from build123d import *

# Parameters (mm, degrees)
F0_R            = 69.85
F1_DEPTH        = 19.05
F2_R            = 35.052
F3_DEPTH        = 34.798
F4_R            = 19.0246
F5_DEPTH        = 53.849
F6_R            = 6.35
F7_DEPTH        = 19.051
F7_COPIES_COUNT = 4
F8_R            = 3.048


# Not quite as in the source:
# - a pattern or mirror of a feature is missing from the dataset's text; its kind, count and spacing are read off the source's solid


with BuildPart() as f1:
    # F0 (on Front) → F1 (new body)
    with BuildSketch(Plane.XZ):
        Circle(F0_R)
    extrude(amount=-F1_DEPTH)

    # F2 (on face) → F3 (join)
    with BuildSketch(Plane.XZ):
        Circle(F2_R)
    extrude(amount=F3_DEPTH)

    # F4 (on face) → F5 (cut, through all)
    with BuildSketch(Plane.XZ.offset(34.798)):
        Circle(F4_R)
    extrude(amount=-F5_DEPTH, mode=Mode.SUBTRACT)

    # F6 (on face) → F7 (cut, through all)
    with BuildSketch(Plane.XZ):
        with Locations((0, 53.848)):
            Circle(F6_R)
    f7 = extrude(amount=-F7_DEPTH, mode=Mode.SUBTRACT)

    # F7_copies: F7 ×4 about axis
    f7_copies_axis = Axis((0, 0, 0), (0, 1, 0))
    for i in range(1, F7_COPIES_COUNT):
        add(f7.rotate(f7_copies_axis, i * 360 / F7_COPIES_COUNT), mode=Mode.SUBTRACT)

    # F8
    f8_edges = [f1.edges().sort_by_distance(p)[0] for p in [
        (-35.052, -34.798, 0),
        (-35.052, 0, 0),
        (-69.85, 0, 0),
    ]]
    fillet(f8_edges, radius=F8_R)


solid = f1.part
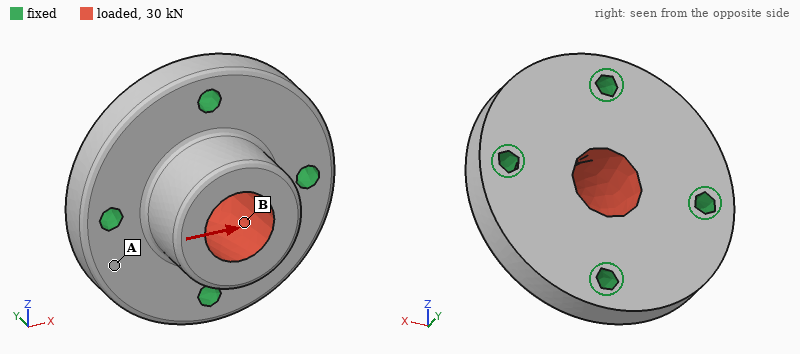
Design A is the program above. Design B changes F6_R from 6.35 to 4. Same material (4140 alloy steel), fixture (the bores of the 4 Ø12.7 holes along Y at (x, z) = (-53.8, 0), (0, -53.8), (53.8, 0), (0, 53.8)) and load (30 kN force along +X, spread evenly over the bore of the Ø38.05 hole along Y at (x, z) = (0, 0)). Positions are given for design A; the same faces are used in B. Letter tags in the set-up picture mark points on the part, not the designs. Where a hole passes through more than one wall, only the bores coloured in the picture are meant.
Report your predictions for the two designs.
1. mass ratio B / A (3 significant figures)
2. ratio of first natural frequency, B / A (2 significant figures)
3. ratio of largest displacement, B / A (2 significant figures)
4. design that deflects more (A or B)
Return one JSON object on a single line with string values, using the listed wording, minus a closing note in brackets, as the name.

{"mass ratio B / A": "1.02", "ratio of first natural frequency, B / A": "0.90", "ratio of largest displacement, B / A": "1.1", "design that deflects more": "B"}
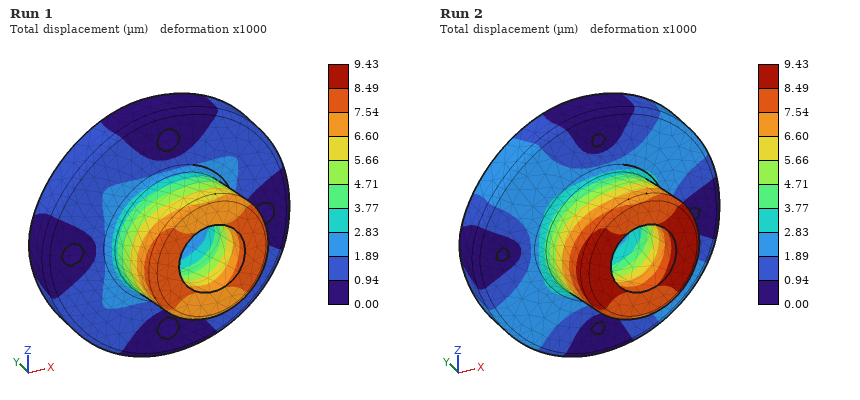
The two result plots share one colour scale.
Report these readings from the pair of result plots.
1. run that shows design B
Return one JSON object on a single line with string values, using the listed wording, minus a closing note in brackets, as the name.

{"run that shows design B": "Run 2"}
